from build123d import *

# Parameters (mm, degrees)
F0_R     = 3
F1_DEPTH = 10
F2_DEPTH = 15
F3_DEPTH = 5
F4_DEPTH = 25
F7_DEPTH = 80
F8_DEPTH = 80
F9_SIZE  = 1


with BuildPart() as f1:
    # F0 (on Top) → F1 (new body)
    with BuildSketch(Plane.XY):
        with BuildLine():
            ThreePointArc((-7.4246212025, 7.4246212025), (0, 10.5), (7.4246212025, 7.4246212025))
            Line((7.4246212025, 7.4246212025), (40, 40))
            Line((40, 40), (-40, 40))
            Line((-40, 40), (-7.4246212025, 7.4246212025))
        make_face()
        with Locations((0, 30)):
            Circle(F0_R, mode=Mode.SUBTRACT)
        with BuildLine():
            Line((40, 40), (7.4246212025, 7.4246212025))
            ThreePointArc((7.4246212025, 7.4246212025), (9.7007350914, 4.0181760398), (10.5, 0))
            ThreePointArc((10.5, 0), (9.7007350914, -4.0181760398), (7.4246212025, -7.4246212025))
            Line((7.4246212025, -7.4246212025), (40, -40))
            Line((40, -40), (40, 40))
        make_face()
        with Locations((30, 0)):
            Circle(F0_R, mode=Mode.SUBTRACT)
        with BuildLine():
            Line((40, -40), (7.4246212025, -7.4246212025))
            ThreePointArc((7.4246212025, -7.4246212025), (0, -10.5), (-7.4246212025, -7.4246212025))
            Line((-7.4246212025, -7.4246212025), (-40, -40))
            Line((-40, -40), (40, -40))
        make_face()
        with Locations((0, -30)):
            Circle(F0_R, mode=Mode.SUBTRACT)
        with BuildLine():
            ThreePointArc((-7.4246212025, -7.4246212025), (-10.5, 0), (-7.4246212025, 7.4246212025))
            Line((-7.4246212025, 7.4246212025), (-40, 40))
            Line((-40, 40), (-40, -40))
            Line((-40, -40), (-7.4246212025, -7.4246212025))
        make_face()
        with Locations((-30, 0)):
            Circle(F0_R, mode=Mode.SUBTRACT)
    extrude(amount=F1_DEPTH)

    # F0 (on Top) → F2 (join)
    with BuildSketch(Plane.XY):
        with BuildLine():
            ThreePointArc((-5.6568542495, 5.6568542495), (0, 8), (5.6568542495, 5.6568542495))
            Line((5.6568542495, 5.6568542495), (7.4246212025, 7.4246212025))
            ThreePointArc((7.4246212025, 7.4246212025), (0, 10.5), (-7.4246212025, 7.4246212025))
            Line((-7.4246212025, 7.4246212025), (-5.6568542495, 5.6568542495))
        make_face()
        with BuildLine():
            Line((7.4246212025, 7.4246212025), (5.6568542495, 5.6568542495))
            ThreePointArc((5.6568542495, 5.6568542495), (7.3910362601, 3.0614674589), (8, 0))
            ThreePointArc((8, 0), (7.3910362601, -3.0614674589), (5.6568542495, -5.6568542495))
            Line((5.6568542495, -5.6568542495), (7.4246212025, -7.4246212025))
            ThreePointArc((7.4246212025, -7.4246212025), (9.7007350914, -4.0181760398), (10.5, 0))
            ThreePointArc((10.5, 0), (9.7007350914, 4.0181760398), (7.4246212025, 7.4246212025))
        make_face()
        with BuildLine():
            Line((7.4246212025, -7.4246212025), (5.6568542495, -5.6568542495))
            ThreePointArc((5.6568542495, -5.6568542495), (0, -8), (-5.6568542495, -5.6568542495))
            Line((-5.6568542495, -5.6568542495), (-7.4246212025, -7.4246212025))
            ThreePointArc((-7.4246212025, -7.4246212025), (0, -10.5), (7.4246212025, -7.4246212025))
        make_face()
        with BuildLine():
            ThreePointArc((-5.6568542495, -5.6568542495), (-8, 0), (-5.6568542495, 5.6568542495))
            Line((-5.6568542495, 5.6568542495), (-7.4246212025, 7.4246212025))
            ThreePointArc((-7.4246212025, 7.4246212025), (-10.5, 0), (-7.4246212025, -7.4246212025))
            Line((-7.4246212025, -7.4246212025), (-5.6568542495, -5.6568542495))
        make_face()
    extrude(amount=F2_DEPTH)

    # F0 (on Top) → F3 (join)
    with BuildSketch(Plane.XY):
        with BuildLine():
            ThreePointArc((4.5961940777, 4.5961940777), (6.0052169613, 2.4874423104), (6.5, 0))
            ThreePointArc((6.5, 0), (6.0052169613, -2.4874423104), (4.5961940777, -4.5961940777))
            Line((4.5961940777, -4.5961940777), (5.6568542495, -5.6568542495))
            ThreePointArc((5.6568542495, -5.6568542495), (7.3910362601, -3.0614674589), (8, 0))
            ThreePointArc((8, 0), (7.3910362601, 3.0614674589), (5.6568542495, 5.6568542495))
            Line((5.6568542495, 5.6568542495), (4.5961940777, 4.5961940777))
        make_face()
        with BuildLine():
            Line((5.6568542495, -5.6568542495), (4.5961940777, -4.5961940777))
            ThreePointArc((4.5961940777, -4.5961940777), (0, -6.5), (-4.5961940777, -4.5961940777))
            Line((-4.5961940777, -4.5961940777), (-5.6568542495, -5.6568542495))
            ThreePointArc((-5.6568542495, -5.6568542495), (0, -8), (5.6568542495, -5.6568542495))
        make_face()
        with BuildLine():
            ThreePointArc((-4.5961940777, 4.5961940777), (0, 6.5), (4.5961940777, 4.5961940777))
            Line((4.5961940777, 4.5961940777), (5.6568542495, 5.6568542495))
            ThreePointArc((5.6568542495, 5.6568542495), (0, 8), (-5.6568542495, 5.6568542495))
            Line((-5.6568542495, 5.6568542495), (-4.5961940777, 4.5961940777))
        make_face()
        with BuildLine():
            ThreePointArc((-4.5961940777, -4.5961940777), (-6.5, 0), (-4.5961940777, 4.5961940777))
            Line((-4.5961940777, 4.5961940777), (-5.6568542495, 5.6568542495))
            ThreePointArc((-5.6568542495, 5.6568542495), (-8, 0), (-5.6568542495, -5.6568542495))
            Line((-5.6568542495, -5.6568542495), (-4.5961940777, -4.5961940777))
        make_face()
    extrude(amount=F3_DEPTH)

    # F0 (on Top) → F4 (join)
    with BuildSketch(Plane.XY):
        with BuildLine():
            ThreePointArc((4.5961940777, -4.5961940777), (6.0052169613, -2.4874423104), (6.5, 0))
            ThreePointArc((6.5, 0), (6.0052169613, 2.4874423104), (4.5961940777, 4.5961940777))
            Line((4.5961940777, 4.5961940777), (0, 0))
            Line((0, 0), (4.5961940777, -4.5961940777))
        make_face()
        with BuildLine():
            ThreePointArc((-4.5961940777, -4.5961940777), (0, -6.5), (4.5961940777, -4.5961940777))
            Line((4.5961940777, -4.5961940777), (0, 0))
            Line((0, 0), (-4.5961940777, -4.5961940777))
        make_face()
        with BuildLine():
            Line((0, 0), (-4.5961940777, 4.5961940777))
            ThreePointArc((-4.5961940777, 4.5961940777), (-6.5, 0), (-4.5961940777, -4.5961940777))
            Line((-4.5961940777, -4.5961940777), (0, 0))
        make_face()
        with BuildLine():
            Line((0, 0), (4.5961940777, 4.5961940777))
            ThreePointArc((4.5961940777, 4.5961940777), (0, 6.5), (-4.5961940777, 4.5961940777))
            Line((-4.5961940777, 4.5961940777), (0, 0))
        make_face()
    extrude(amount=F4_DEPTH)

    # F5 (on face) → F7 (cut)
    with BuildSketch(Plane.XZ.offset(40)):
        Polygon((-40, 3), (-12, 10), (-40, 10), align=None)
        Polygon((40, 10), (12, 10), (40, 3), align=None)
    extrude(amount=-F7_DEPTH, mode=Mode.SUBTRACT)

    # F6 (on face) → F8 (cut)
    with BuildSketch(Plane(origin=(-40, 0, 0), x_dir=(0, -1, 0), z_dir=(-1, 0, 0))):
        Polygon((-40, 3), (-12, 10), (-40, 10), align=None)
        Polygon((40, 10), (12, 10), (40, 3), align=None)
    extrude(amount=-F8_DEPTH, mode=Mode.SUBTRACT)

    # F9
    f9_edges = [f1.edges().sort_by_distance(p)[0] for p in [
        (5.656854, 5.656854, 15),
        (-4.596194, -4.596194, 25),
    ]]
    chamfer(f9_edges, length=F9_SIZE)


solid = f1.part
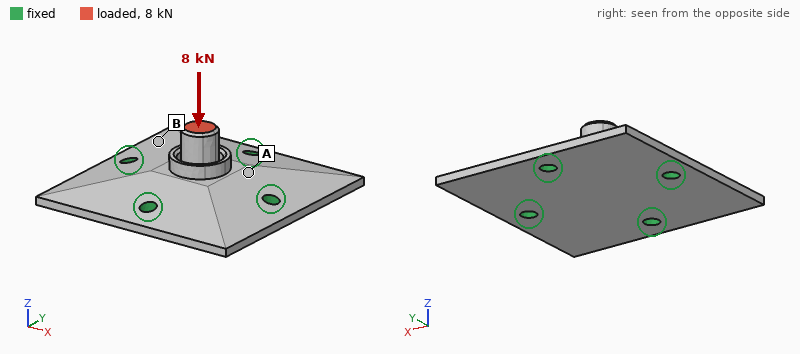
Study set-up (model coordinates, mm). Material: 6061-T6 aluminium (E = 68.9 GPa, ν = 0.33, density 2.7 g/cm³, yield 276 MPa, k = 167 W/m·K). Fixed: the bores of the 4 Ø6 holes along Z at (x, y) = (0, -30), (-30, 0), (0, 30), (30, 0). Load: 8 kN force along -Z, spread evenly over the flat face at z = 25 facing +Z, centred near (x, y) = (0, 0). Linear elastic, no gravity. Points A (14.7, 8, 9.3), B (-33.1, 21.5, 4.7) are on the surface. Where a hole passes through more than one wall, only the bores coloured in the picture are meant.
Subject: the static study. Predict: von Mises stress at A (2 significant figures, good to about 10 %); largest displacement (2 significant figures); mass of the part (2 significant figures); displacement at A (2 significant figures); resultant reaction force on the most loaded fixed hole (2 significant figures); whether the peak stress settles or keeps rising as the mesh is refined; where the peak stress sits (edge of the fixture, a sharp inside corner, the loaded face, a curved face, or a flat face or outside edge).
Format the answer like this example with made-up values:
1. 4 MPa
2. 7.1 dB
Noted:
1. 42 MPa
2. 74 µm
3. 110 g
4. 28 µm
5. 2.4 kN
6. keeps rising
7. edge of the fixture
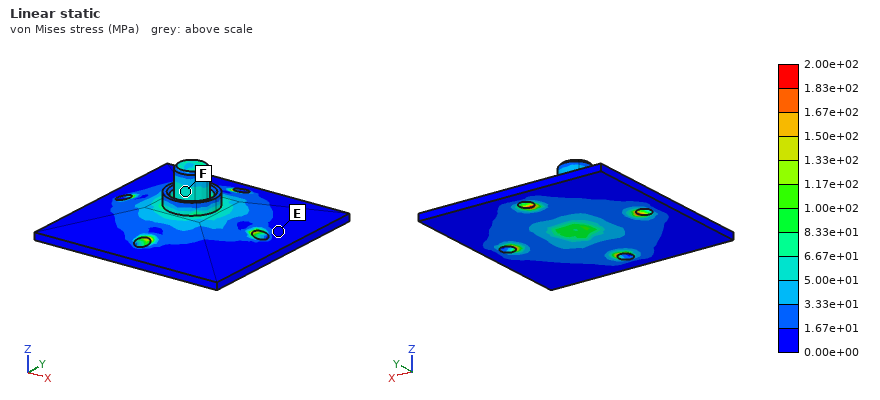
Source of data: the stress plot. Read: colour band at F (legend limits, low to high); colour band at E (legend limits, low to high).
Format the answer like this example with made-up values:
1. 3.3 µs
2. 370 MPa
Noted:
1. 5.00e+01 to 6.67e+01 MPa
2. 0.00e+00 to 1.67e+01 MPa
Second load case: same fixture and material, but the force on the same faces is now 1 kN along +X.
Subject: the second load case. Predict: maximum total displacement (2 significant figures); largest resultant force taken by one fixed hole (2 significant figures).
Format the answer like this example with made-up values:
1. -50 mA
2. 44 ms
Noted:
1. 69 µm
2. 600 N
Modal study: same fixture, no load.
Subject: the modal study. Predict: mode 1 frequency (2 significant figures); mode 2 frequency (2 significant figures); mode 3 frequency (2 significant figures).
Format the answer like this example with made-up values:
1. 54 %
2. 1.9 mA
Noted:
1. 6800 Hz
2. 7000 Hz
3. 7100 Hz
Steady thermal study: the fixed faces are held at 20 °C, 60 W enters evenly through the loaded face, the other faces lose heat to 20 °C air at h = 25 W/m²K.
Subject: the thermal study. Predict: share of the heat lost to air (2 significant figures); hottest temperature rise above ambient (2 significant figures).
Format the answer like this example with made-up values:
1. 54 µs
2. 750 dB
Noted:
1. 4.2 %
2. 76 K
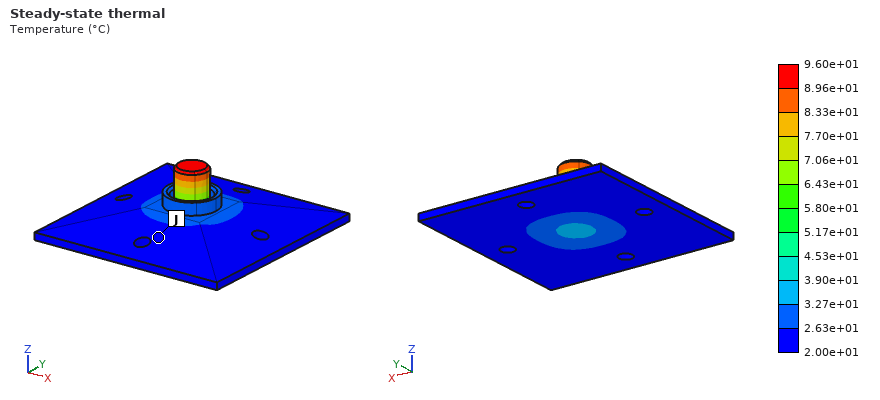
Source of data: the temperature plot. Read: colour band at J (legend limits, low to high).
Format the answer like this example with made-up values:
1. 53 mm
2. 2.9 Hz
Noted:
1. 2.00e+01 to 2.63e+01 °C
